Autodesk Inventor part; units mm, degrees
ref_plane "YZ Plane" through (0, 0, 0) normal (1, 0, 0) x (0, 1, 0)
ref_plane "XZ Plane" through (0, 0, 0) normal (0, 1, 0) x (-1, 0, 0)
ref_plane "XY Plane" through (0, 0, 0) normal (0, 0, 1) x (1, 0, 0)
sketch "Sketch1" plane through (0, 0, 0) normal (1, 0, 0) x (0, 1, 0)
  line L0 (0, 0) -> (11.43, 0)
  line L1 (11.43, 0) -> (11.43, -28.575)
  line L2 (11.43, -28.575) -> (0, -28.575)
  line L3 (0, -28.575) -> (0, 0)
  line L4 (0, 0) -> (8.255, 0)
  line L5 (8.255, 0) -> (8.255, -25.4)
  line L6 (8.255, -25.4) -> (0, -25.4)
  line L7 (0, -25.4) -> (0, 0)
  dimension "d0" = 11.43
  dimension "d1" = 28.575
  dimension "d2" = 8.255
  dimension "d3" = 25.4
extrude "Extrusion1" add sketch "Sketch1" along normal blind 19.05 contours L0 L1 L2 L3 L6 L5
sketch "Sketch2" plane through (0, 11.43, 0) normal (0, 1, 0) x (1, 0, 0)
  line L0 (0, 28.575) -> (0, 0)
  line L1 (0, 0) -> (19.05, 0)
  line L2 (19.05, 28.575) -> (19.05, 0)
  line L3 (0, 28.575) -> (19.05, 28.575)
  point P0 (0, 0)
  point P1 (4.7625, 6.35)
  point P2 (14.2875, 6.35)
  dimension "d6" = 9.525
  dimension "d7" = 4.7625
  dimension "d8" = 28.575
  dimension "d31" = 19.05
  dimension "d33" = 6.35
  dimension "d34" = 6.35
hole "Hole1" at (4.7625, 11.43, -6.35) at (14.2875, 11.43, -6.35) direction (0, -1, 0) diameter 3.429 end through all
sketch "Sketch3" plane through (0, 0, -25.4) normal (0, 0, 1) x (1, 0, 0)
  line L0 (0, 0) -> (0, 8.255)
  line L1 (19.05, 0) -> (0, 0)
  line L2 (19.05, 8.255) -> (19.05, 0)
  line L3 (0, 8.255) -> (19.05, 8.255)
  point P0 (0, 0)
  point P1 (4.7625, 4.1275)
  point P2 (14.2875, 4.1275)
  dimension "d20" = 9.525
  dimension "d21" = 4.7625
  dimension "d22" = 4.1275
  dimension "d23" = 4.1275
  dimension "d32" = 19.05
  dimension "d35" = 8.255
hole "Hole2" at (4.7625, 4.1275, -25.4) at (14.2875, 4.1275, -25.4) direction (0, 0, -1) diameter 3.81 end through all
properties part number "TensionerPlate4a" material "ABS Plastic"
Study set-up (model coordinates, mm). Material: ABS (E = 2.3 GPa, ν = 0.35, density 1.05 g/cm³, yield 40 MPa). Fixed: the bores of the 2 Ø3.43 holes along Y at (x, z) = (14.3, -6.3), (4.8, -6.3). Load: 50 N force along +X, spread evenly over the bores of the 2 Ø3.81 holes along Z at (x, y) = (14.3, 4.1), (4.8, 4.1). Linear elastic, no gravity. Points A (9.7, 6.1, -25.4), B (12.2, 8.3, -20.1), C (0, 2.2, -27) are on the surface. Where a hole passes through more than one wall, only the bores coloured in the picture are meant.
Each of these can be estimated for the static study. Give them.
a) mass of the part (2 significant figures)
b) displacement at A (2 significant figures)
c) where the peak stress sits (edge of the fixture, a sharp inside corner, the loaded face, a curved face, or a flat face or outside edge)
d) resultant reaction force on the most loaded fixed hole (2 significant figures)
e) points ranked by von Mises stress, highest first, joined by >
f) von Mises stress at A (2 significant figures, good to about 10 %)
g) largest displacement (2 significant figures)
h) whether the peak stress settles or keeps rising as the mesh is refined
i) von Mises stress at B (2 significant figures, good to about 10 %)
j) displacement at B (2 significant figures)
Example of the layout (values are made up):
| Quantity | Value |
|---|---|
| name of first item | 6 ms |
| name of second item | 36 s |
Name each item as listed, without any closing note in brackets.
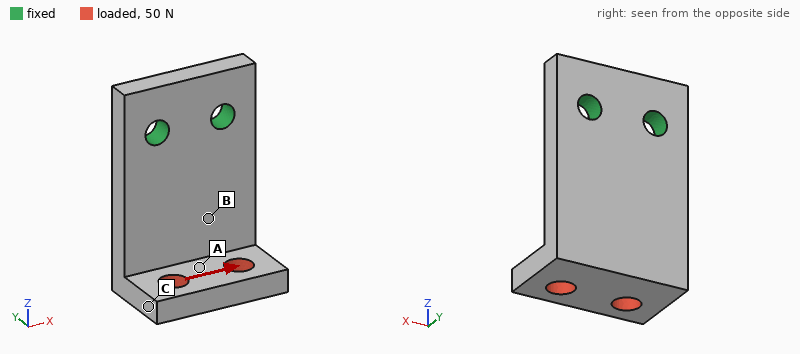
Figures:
| Quantity | Value |
|---|---|
| mass of the part | 2.2 g |
| displacement at A | 0.15 mm |
| where the peak stress sits | edge of the fixture |
| resultant reaction force on the most loaded fixed hole | 91 N |
| points ranked by von Mises stress, highest first, joined by > | B > A > C |
| von Mises stress at A | 4.1 MPa |
| largest displacement | 0.39 mm |
| whether the peak stress settles or keeps rising as the mesh is refined | keeps rising |
| von Mises stress at B | 8.8 MPa |
| displacement at B | 0.074 mm |
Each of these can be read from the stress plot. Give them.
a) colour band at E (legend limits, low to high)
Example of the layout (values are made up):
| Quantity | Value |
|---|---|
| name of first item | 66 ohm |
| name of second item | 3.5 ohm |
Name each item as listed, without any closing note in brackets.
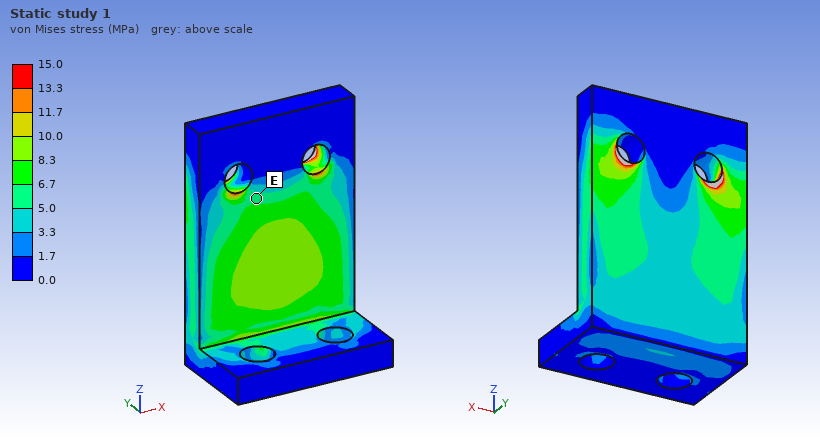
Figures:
| Quantity | Value |
|---|---|
| colour band at E | 5.0 to 6.7 MPa |
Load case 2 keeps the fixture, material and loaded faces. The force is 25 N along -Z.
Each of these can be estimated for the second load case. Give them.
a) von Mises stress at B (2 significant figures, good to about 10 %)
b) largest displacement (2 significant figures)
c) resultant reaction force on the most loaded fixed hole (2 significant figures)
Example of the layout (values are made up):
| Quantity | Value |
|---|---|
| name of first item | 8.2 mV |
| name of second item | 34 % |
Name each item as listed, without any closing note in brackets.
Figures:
| Quantity | Value |
|---|---|
| von Mises stress at B | 4.6 MPa |
| largest displacement | 0.37 mm |
| resultant reaction force on the most loaded fixed hole | 13 N |
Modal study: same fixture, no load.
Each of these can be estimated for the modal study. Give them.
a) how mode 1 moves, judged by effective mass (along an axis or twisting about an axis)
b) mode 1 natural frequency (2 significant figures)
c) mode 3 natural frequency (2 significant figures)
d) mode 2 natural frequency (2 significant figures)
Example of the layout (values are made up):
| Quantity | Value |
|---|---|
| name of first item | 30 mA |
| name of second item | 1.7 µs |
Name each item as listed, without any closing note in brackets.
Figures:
| Quantity | Value |
|---|---|
| how mode 1 moves, judged by effective mass | along Y |
| mode 1 natural frequency | 1100 Hz |
| mode 3 natural frequency | 4500 Hz |
| mode 2 natural frequency | 2400 Hz |
